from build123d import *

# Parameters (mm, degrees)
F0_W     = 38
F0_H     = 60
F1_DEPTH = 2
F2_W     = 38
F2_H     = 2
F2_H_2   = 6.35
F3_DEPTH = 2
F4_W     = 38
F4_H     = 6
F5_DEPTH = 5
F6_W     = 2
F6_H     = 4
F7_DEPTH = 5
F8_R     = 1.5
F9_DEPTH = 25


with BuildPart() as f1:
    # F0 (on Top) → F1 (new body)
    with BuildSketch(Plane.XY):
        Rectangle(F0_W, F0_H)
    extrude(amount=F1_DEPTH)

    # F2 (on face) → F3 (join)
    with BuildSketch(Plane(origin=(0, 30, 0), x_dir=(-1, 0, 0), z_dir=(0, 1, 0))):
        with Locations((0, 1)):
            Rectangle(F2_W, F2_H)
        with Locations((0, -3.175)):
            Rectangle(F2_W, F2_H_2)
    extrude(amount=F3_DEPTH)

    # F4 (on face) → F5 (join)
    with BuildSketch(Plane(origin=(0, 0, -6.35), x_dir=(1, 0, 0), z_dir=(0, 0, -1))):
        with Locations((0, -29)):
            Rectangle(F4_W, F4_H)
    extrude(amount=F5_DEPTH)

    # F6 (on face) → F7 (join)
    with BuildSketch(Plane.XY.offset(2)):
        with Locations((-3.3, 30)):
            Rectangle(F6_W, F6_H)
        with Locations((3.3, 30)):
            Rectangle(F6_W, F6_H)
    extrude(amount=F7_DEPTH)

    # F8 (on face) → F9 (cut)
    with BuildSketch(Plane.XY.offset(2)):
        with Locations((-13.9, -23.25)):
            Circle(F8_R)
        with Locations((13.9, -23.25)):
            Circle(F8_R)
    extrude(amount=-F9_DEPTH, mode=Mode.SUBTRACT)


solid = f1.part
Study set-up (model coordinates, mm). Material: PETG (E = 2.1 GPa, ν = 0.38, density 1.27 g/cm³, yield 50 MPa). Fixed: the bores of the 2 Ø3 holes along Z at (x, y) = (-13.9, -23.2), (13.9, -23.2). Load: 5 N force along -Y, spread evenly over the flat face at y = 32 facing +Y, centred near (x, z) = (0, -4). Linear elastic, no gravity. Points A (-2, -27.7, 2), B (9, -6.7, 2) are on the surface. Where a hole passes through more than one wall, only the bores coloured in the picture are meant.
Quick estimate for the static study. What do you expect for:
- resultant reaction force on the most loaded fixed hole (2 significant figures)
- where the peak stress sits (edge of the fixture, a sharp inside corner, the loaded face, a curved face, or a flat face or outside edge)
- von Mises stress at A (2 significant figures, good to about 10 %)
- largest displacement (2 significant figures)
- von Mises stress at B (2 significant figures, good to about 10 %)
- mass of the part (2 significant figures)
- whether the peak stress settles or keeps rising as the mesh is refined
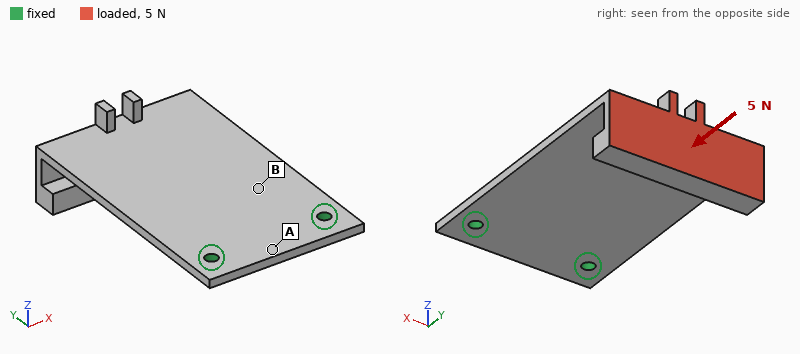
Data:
2.5 N
edge of the fixture
0.27 MPa
0.83 mm
0.92 MPa
8.1 g
keeps rising
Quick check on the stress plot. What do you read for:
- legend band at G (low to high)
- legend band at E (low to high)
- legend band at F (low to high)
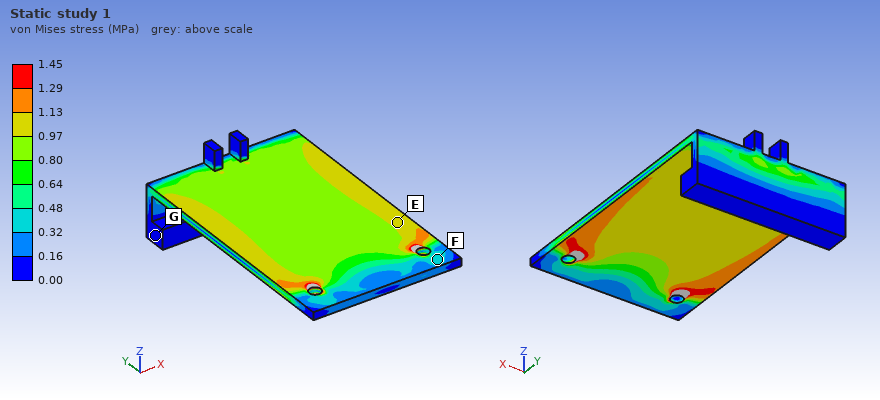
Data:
0.00 to 0.16 MPa
0.97 to 1.13 MPa
0.32 to 0.48 MPa
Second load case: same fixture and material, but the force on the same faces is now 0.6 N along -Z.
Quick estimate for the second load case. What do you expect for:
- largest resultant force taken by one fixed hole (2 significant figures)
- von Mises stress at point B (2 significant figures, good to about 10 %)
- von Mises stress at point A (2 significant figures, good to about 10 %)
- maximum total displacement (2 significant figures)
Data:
0.30 N
0.86 MPa
0.27 MPa
0.68 mm
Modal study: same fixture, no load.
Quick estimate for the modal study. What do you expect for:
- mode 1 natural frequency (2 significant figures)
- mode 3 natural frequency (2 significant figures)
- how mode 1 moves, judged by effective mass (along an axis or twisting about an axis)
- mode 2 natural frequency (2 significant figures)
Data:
85 Hz
540 Hz
along Z
280 Hz
